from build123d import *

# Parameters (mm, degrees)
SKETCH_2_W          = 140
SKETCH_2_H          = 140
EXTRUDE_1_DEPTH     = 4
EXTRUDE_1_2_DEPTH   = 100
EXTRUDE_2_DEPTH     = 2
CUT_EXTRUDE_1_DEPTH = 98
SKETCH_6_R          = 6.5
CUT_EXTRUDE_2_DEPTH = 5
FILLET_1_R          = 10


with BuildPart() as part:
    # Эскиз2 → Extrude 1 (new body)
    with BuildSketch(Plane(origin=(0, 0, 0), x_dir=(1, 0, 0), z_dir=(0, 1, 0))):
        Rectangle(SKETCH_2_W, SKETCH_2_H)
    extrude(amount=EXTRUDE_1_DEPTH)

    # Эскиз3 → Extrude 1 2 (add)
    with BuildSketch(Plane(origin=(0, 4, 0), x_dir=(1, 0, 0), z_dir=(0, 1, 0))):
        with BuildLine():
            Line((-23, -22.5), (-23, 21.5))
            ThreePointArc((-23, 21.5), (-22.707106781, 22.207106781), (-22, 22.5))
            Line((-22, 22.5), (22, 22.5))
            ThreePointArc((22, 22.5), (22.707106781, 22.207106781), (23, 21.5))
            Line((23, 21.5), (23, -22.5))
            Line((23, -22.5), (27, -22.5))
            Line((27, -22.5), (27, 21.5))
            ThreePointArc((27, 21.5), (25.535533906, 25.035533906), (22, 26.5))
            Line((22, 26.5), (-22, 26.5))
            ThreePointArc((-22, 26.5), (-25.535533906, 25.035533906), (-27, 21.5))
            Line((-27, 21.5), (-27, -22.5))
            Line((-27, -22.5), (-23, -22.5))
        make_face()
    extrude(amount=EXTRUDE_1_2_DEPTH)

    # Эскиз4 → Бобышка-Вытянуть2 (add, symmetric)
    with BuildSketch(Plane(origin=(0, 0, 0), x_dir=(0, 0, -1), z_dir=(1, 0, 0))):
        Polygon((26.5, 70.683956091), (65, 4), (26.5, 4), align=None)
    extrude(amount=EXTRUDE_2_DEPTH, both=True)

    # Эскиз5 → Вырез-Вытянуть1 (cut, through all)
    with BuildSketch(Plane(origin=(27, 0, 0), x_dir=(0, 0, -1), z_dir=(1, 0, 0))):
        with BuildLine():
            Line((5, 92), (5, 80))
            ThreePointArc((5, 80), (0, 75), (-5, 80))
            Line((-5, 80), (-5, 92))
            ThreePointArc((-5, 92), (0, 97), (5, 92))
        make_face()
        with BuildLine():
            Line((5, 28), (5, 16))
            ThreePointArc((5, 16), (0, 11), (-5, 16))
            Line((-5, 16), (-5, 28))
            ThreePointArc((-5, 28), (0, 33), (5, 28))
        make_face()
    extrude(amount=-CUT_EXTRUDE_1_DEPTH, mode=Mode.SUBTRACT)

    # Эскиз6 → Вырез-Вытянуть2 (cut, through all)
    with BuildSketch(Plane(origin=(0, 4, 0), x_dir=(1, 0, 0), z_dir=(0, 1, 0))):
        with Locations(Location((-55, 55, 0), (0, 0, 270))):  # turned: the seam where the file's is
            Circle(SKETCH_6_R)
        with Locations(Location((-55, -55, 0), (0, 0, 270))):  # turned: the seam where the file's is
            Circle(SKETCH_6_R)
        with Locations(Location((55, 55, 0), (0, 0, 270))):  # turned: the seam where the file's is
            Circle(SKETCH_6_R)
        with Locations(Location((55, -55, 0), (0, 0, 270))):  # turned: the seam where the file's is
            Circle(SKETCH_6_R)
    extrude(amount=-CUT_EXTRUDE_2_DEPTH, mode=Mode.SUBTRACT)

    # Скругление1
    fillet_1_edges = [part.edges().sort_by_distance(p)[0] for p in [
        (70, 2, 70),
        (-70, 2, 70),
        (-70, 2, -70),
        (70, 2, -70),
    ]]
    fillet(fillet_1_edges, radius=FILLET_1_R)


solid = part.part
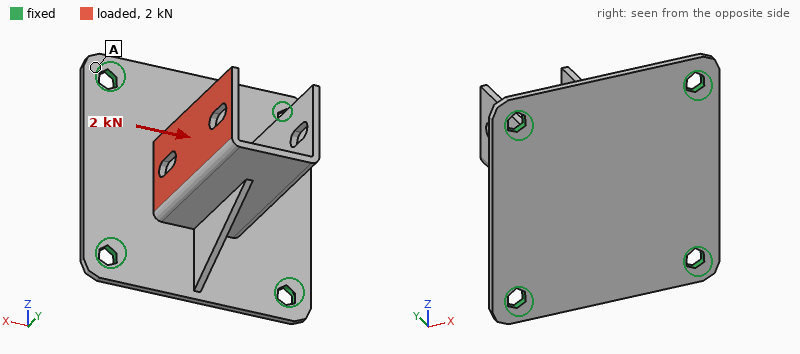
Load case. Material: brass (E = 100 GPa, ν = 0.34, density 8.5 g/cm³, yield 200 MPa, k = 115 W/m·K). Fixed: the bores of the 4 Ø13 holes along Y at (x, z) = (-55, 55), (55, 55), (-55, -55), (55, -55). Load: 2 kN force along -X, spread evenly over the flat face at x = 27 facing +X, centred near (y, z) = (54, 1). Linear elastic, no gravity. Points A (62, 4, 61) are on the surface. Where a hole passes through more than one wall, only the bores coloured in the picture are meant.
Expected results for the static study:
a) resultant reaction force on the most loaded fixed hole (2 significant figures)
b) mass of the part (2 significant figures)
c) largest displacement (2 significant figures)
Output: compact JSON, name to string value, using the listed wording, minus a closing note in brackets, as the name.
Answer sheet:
{"resultant reaction force on the most loaded fixed hole": "1.1 kN", "mass of the part": "1.1 kg", "largest displacement": "1.7 mm"}
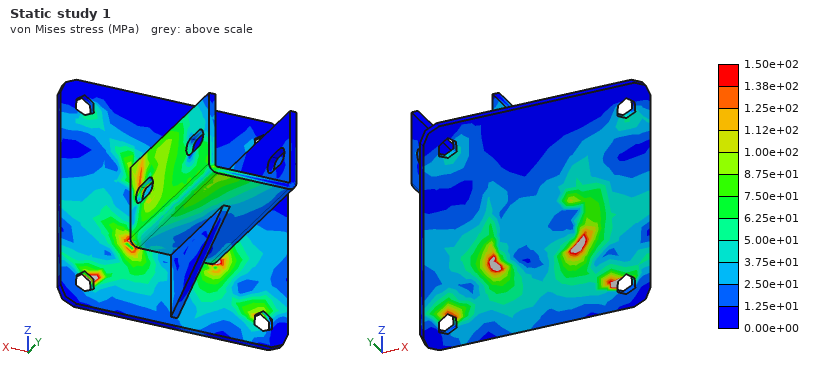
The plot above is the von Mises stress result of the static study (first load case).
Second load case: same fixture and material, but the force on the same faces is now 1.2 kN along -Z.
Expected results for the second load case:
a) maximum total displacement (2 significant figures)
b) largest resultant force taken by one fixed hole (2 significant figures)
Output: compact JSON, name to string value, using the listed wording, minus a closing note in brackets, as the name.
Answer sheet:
{"maximum total displacement": "0.46 mm", "largest resultant force taken by one fixed hole": "630 N"}
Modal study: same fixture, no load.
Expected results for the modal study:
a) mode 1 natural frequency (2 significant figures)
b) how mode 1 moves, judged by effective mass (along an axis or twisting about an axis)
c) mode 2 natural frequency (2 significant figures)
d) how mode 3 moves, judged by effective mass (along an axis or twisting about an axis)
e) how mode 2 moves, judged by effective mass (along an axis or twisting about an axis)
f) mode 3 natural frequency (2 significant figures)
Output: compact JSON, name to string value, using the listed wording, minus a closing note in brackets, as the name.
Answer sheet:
{"mode 1 natural frequency": "440 Hz", "how mode 1 moves, judged by effective mass": "along X", "mode 2 natural frequency": "590 Hz", "how mode 3 moves, judged by effective mass": "along Y", "how mode 2 moves, judged by effective mass": "along Z", "mode 3 natural frequency": "720 Hz"}
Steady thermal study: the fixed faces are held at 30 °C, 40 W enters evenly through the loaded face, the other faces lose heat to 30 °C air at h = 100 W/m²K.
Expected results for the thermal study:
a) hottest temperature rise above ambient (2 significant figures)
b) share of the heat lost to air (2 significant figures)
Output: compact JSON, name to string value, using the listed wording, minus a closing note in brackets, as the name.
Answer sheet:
{"hottest temperature rise above ambient": "31 K", "share of the heat lost to air": "83 %"}
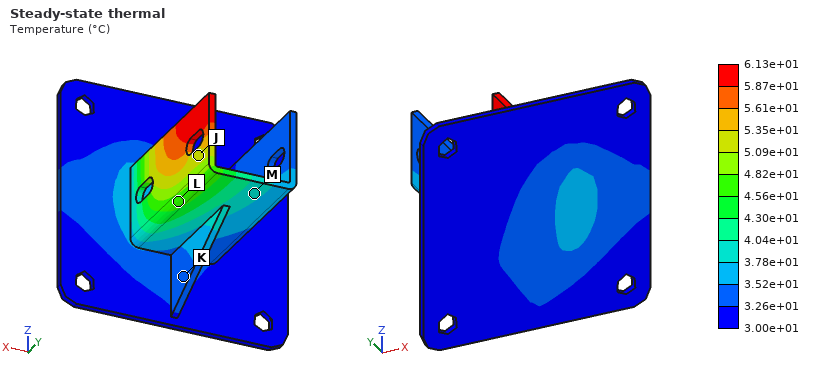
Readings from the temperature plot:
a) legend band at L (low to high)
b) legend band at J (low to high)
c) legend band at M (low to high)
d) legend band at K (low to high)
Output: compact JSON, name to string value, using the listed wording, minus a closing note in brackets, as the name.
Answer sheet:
{"legend band at L": "4.56e+01 to 4.82e+01 °C", "legend band at J": "5.09e+01 to 5.35e+01 °C", "legend band at M": "3.78e+01 to 4.04e+01 °C", "legend band at K": "3.26e+01 to 3.52e+01 °C"}
